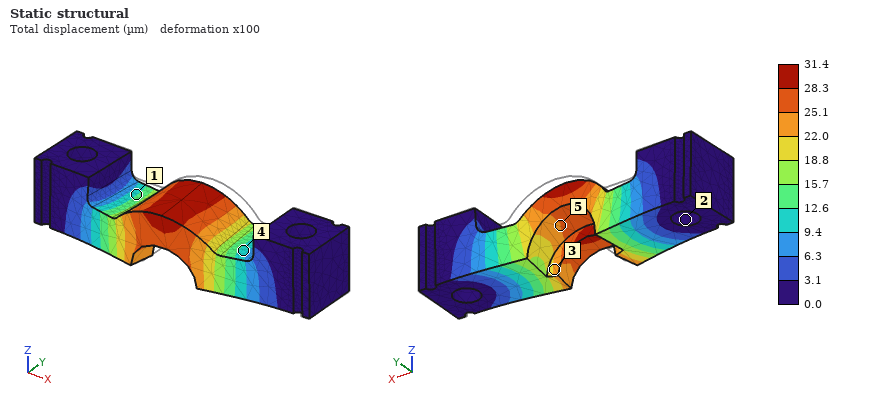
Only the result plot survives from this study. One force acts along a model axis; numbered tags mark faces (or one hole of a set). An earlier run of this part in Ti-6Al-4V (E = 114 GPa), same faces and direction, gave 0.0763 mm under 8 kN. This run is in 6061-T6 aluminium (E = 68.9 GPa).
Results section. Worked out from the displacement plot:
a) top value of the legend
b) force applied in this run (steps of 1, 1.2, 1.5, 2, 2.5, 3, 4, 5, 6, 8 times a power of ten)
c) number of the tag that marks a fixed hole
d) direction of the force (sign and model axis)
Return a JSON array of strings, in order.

["31.4 µm", "2 kN", "2", "-Y"]
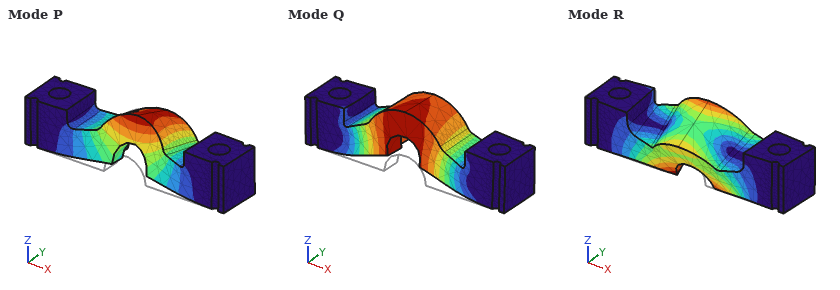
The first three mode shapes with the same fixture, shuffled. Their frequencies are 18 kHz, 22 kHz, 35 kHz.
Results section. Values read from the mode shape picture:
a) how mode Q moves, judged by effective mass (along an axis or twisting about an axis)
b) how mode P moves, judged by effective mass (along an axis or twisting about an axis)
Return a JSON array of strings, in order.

["along Z", "along Y"]
